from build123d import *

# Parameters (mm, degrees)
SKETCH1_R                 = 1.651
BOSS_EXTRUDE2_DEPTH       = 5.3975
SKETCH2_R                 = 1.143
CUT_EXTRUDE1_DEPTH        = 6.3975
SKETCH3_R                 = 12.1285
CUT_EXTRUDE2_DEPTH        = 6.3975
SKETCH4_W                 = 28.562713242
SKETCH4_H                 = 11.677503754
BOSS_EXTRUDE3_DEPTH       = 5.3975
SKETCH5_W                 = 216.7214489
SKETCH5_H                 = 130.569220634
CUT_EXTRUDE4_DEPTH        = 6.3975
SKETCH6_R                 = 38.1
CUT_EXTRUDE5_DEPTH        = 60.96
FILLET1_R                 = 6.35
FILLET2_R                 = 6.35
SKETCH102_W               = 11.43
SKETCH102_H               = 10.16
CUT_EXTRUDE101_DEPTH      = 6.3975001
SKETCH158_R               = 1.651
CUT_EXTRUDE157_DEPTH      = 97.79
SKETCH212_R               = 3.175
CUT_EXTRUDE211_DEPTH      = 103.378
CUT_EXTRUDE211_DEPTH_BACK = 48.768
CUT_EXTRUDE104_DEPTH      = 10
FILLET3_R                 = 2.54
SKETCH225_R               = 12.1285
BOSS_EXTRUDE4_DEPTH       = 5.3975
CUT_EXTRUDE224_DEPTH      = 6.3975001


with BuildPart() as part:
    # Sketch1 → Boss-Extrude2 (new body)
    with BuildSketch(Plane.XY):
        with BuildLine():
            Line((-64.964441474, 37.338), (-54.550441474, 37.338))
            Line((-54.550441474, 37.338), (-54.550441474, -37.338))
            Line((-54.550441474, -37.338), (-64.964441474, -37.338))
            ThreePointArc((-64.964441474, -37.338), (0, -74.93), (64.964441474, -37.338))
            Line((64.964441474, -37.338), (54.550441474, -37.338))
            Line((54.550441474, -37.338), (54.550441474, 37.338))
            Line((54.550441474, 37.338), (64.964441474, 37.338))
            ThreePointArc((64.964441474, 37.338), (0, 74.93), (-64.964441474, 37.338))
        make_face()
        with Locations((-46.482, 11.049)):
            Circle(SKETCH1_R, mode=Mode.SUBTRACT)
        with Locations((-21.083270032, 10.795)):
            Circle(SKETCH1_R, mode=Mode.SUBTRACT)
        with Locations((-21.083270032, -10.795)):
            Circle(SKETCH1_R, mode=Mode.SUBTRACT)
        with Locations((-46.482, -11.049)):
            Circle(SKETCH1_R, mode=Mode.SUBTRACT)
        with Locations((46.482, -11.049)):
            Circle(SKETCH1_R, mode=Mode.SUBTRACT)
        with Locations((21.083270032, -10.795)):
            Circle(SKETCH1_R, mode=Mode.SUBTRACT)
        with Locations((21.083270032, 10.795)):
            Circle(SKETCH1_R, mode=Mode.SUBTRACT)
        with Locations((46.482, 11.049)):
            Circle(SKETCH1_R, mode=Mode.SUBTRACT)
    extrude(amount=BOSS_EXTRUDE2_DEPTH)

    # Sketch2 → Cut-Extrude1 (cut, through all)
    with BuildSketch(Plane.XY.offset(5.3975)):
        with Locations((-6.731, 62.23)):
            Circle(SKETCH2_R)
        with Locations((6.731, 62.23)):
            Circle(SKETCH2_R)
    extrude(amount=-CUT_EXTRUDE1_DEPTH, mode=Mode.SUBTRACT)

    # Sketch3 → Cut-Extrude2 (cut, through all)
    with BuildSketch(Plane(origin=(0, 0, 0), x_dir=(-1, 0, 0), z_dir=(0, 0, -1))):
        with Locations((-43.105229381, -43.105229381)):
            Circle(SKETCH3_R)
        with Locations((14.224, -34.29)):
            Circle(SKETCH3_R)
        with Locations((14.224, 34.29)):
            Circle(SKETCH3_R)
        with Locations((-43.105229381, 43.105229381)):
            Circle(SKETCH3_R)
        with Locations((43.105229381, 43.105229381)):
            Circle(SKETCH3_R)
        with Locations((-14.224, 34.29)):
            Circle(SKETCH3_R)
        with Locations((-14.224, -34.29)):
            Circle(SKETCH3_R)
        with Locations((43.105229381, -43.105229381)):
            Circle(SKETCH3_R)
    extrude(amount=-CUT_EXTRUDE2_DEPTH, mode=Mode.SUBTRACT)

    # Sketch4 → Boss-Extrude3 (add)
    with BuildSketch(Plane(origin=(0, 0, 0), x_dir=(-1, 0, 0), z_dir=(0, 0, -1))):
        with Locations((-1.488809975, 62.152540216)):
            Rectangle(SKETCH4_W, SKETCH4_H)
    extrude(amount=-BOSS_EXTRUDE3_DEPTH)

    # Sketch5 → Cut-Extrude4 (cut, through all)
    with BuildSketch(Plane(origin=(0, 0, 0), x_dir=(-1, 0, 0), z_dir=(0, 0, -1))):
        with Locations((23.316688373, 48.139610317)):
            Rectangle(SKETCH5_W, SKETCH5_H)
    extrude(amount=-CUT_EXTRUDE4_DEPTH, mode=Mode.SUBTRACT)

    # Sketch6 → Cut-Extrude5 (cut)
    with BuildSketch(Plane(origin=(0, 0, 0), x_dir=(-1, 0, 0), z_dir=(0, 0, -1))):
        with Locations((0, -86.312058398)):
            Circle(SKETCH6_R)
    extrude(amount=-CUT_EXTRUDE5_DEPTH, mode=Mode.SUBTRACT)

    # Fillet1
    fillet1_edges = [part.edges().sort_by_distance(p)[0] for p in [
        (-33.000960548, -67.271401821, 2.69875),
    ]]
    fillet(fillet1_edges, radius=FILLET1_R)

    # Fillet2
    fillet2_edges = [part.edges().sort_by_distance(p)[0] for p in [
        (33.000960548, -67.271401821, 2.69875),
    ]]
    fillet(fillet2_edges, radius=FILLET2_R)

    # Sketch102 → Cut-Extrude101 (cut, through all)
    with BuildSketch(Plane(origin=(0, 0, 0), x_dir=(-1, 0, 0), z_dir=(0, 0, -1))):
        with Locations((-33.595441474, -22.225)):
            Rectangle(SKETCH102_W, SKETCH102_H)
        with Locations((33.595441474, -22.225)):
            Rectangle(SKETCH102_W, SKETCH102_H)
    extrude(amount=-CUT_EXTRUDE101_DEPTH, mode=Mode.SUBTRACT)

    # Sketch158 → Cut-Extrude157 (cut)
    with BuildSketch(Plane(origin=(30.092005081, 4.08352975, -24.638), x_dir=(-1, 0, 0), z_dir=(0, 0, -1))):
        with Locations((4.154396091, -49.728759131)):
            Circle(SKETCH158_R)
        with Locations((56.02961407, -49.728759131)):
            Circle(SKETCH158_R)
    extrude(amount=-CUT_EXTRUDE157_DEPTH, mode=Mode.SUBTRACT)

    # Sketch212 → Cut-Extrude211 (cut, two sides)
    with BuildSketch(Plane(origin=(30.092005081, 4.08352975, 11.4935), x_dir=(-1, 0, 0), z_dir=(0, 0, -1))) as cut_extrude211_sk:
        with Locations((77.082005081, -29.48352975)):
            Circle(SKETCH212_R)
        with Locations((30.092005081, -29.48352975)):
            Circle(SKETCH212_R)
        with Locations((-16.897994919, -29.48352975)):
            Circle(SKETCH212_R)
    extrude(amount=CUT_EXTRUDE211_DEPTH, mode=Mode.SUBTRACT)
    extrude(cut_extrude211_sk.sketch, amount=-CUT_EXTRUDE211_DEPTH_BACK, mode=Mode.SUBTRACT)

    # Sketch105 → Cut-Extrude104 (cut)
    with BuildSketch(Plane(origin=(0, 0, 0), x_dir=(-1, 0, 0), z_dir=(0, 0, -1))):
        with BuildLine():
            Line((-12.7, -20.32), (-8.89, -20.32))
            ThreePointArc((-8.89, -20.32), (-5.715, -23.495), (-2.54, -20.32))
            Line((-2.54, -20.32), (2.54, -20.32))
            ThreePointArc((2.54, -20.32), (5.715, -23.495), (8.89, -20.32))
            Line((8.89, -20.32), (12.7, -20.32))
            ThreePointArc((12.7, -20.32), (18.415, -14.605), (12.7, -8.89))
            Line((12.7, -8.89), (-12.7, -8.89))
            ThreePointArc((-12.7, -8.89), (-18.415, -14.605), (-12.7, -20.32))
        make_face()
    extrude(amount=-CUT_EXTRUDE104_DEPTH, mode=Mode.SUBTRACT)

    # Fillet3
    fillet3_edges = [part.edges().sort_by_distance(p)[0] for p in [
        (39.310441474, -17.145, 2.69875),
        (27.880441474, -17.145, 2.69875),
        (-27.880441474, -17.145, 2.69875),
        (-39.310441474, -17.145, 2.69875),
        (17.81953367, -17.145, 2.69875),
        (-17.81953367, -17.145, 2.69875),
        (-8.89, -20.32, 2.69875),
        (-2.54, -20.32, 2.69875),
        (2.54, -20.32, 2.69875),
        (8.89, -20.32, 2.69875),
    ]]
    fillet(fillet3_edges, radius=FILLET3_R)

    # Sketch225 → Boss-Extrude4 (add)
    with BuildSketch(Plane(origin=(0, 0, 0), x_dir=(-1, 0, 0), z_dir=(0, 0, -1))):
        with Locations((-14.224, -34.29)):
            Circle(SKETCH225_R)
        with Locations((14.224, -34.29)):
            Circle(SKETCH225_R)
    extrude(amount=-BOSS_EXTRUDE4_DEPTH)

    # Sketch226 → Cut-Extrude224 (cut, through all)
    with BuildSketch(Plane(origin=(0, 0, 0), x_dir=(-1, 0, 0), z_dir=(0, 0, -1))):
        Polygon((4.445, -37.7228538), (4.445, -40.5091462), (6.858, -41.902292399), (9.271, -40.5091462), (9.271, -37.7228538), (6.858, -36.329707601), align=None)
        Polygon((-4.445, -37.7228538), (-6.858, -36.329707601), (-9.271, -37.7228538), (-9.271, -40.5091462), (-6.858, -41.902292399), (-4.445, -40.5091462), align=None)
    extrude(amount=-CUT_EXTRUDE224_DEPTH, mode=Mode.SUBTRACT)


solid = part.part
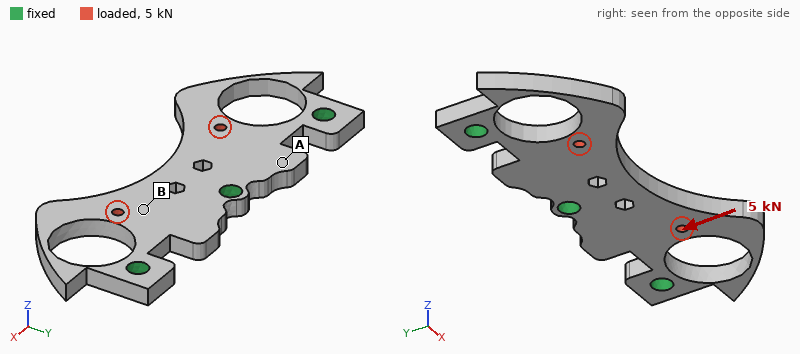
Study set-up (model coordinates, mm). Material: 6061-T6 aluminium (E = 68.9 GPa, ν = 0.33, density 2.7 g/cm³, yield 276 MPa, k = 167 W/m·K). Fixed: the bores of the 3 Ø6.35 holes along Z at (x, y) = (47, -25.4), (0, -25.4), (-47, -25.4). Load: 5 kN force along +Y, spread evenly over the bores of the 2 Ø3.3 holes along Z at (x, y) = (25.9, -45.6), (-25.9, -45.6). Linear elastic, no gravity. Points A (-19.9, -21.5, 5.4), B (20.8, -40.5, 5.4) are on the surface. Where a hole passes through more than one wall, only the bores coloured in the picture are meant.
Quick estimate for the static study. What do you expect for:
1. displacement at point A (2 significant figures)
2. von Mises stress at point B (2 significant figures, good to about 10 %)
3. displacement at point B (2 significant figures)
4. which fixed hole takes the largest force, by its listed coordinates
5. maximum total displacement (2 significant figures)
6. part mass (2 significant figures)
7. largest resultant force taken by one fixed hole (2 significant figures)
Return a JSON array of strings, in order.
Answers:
["19 µm", "25 MPa", "20 µm", "(0, -25.4)", "32 µm", "43 g", "3.1 kN"]
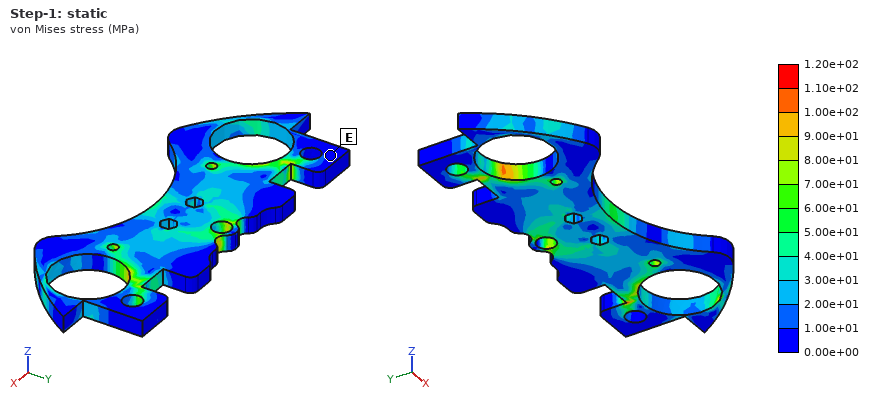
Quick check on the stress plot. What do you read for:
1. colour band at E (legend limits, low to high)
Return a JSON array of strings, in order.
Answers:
["0.00e+00 to 1.00e+01 MPa"]
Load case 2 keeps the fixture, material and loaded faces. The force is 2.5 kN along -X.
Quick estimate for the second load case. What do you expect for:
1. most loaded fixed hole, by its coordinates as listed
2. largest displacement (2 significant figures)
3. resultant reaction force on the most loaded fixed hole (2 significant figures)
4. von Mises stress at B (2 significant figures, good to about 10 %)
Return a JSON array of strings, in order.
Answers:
["(0, -25.4)", "18 µm", "1.2 kN", "16 MPa"]
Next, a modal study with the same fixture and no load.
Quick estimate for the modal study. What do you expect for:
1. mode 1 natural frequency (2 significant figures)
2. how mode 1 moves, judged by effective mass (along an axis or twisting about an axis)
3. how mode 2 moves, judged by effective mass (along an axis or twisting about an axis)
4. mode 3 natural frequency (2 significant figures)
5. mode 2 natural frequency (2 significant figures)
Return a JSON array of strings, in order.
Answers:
["2700 Hz", "along Z", "twisting about Y", "6600 Hz", "3000 Hz"]
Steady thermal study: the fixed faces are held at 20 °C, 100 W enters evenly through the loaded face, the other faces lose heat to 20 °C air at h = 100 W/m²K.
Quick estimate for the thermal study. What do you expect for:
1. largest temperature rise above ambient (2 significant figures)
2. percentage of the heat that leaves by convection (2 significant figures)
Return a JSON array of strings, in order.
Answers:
["64 K", "24 %"]
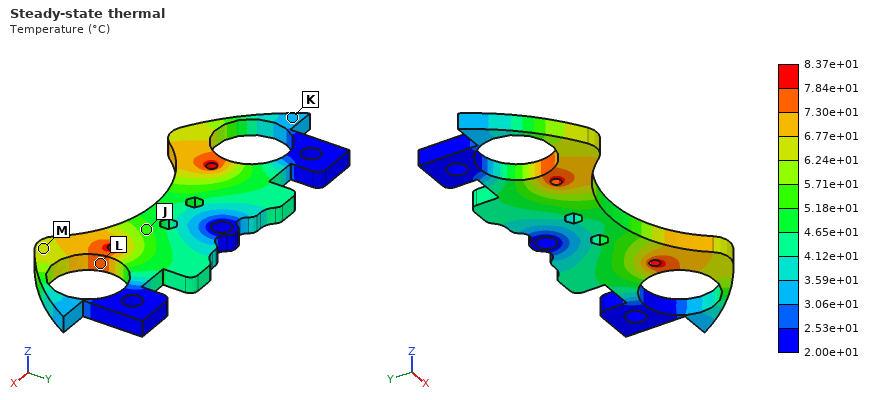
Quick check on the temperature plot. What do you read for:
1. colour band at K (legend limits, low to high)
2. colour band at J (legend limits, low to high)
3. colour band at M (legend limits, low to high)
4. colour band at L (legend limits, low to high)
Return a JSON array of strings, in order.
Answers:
["3.06e+01 to 3.59e+01 °C", "5.18e+01 to 5.71e+01 °C", "6.24e+01 to 6.77e+01 °C", "7.30e+01 to 7.84e+01 °C"]
